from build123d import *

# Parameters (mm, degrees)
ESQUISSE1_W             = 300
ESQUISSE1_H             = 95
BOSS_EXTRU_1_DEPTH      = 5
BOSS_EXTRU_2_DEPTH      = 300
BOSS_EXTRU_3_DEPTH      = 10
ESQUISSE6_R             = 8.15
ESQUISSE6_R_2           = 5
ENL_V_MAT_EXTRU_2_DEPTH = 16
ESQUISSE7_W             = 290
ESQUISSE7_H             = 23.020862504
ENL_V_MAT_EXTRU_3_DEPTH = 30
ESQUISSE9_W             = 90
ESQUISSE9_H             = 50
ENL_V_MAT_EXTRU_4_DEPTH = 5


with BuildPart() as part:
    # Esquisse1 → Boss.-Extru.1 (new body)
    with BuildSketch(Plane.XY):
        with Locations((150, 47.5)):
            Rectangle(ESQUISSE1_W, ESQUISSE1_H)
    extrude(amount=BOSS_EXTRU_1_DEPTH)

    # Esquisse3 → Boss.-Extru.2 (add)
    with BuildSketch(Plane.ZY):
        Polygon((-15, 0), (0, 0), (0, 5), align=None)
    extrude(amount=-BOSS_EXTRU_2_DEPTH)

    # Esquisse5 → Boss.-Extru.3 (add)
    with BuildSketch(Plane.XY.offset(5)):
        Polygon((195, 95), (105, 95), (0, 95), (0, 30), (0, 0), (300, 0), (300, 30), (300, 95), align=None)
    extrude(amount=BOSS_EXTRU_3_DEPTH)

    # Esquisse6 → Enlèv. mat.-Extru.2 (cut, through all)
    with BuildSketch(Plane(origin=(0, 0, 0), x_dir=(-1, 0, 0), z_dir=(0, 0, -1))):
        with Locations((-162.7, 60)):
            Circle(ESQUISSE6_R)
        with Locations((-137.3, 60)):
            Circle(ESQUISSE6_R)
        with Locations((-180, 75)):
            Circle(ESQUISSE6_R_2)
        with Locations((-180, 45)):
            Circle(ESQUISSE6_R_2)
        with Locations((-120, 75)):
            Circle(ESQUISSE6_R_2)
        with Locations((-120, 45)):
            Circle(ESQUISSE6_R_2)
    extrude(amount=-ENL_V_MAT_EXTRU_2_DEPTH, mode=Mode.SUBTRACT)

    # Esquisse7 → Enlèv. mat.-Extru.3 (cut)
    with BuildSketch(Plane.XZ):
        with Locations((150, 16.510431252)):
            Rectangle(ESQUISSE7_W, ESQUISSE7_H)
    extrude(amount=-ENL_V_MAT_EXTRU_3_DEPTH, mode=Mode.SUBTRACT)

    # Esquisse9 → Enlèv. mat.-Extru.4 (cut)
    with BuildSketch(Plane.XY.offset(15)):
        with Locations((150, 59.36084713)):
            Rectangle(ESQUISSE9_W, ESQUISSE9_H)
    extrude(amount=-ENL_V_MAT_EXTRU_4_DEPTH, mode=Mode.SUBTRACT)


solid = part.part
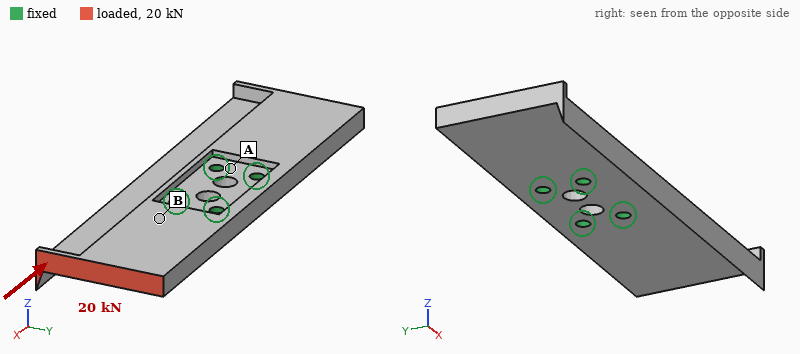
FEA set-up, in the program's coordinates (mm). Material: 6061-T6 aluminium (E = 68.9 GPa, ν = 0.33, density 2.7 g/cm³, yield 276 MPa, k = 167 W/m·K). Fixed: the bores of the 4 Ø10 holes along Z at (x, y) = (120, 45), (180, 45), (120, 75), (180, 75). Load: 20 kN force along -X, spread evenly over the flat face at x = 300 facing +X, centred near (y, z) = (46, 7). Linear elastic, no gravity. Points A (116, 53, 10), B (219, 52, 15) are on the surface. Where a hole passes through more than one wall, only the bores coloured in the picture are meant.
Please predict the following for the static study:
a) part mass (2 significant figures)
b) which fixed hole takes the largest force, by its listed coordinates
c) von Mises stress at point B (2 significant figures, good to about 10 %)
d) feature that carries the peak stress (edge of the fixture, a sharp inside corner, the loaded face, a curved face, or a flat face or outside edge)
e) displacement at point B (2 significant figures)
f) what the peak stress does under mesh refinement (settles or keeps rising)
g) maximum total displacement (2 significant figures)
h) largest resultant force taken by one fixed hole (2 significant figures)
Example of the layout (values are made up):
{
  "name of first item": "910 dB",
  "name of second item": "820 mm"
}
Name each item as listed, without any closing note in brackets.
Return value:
{
  "part mass": "870 g",
  "which fixed hole takes the largest force, by its listed coordinates": "(180, 45)",
  "von Mises stress at point B": "26 MPa",
  "feature that carries the peak stress": "edge of the fixture",
  "displacement at point B": "0.059 mm",
  "what the peak stress does under mesh refinement": "keeps rising",
  "maximum total displacement": "0.39 mm",
  "largest resultant force taken by one fixed hole": "13 kN"
}
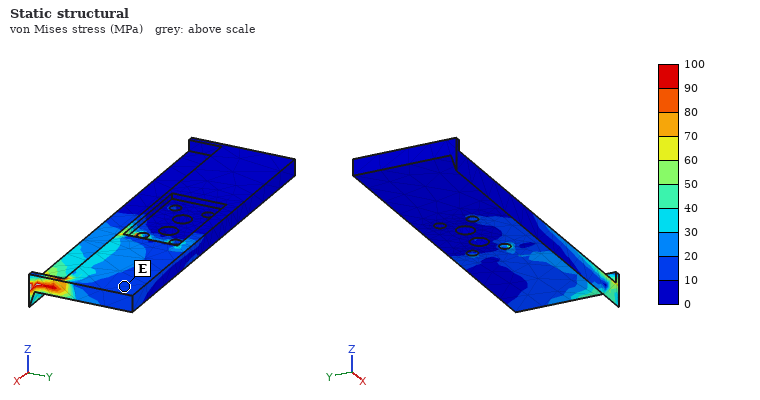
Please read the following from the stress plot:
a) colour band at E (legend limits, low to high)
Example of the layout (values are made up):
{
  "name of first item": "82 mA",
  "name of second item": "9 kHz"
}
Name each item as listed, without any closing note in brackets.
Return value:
{
  "colour band at E": "10 to 20 MPa"
}
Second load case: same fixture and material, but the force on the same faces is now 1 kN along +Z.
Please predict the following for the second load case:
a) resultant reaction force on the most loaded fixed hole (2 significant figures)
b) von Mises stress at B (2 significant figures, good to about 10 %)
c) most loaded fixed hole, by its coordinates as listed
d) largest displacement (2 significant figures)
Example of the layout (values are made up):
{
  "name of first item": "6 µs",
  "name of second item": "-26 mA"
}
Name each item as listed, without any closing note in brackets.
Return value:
{
  "resultant reaction force on the most loaded fixed hole": "1.7 kN",
  "von Mises stress at B": "25 MPa",
  "most loaded fixed hole, by its coordinates as listed": "(180, 45)",
  "largest displacement": "0.62 mm"
}
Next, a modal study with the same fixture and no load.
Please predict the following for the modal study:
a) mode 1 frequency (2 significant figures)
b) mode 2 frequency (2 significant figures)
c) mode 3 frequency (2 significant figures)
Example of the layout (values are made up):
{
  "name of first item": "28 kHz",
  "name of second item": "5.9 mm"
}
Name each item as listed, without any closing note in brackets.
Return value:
{
  "mode 1 frequency": "660 Hz",
  "mode 2 frequency": "660 Hz",
  "mode 3 frequency": "1800 Hz"
}
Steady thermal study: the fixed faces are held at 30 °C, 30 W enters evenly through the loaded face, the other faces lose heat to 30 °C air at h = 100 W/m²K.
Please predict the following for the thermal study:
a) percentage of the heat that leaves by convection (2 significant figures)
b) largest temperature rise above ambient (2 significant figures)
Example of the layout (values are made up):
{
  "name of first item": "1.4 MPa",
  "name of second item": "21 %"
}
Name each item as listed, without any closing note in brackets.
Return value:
{
  "percentage of the heat that leaves by convection": "57 %",
  "largest temperature rise above ambient": "15 K"
}
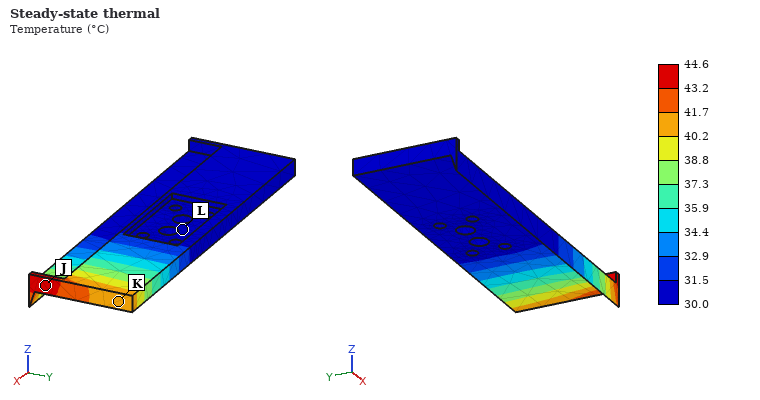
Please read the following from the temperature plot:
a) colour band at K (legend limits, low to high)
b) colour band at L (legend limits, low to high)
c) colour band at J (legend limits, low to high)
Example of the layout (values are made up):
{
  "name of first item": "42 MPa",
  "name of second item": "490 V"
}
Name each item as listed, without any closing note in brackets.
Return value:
{
  "colour band at K": "40.2 to 41.7 °C",
  "colour band at L": "30.0 to 31.5 °C",
  "colour band at J": "43.2 to 44.6 °C"
}
